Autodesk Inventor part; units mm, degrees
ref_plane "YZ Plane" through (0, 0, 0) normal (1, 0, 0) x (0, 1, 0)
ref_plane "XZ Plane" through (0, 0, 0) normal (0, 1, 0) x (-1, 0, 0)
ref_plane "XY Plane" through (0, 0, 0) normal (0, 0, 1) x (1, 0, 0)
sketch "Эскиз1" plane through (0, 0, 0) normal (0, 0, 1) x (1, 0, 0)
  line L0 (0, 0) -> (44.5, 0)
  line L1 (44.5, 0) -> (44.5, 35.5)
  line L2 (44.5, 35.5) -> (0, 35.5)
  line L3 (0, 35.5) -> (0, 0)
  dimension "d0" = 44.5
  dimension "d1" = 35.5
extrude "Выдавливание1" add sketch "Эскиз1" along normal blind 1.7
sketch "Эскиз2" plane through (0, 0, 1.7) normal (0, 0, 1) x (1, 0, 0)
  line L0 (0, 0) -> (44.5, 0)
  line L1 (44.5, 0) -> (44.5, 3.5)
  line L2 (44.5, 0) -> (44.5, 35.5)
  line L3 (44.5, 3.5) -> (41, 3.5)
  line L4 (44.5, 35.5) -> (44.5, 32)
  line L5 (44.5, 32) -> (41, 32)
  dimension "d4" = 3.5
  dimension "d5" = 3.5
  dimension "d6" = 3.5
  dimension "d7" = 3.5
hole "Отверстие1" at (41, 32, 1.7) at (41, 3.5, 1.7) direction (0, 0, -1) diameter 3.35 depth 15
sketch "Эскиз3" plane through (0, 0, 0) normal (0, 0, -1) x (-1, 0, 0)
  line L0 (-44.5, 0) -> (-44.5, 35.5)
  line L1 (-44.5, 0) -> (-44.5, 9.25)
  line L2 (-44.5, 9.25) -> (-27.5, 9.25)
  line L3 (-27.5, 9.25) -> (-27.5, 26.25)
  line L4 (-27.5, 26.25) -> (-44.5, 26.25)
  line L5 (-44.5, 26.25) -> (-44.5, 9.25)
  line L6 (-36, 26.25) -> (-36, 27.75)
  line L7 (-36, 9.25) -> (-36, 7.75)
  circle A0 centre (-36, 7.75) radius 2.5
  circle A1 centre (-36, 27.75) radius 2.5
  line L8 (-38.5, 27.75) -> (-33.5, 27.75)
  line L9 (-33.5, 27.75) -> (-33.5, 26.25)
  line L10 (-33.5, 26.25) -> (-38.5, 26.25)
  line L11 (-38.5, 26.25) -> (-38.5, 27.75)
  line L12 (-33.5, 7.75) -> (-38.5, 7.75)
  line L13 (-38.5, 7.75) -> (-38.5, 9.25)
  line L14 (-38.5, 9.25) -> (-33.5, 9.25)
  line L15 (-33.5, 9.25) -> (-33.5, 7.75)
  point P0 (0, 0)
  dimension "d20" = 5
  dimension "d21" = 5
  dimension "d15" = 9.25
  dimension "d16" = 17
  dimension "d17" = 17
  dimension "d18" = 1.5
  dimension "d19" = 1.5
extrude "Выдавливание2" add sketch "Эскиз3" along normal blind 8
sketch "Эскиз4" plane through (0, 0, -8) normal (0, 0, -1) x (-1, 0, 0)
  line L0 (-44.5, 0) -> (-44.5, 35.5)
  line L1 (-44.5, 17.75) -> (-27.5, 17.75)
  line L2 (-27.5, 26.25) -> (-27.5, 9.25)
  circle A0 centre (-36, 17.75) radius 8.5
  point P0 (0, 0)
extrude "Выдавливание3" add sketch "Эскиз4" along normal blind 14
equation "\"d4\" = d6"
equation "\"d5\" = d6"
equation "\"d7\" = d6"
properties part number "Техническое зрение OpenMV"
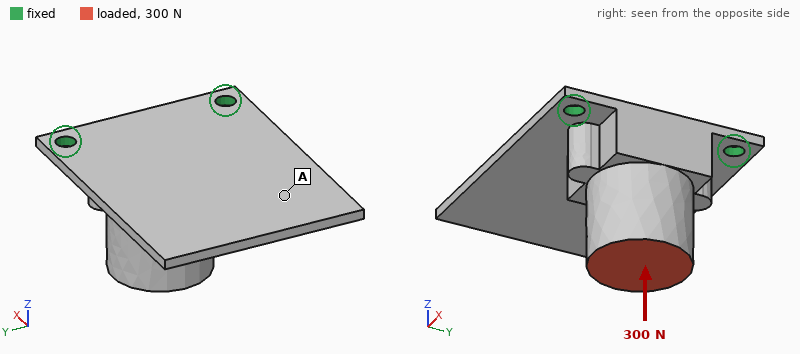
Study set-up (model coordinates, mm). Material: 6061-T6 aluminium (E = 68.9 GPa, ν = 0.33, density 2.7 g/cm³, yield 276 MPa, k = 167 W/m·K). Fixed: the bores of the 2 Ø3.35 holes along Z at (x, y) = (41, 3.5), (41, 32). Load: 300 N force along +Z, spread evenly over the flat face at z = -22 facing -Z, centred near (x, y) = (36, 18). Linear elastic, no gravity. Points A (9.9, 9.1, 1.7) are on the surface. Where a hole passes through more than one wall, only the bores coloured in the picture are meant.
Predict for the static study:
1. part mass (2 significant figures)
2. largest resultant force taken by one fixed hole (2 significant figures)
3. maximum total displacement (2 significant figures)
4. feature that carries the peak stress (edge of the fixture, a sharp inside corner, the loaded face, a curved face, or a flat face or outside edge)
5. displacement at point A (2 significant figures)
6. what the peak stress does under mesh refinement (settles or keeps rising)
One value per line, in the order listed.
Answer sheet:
23 g
160 N
0.13 mm
edge of the fixture
0.10 mm
keeps rising
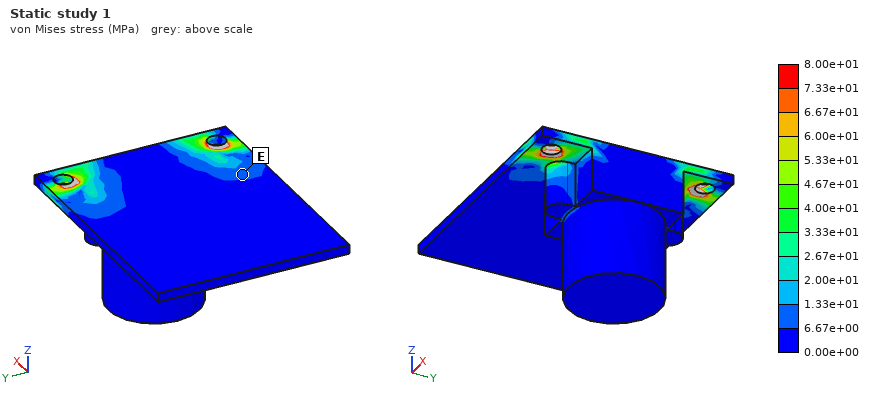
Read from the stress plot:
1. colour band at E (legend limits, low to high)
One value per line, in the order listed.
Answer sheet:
6.67e+00 to 1.33e+01 MPa
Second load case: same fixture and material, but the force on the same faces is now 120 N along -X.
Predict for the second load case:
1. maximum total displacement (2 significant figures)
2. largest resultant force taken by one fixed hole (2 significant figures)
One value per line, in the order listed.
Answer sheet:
0.33 mm
79 N
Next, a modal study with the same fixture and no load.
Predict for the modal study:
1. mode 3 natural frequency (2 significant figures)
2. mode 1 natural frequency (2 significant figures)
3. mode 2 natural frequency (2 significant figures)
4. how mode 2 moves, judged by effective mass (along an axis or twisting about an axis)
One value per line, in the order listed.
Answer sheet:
3100 Hz
1000 Hz
2600 Hz
along X
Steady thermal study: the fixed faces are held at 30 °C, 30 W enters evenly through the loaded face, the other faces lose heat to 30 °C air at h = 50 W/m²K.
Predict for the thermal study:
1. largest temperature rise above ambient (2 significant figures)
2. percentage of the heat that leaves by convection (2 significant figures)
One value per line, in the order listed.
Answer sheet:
38 K
16 %
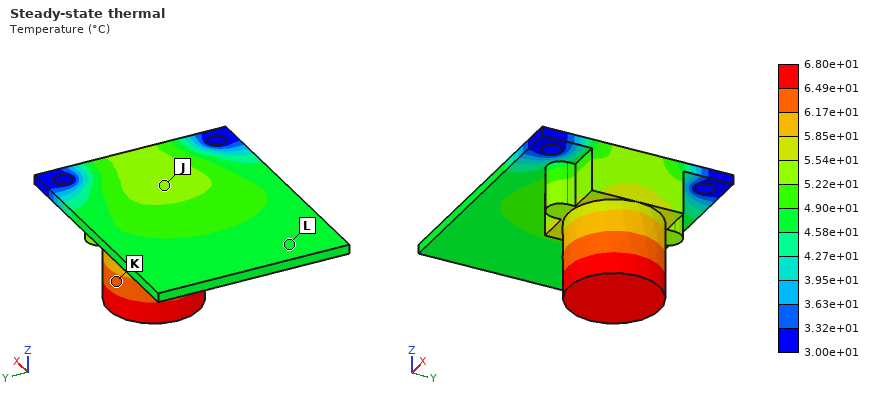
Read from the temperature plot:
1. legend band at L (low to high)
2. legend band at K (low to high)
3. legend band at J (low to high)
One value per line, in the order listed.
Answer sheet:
4.58e+01 to 4.90e+01 °C
6.17e+01 to 6.49e+01 °C
5.22e+01 to 5.54e+01 °C
